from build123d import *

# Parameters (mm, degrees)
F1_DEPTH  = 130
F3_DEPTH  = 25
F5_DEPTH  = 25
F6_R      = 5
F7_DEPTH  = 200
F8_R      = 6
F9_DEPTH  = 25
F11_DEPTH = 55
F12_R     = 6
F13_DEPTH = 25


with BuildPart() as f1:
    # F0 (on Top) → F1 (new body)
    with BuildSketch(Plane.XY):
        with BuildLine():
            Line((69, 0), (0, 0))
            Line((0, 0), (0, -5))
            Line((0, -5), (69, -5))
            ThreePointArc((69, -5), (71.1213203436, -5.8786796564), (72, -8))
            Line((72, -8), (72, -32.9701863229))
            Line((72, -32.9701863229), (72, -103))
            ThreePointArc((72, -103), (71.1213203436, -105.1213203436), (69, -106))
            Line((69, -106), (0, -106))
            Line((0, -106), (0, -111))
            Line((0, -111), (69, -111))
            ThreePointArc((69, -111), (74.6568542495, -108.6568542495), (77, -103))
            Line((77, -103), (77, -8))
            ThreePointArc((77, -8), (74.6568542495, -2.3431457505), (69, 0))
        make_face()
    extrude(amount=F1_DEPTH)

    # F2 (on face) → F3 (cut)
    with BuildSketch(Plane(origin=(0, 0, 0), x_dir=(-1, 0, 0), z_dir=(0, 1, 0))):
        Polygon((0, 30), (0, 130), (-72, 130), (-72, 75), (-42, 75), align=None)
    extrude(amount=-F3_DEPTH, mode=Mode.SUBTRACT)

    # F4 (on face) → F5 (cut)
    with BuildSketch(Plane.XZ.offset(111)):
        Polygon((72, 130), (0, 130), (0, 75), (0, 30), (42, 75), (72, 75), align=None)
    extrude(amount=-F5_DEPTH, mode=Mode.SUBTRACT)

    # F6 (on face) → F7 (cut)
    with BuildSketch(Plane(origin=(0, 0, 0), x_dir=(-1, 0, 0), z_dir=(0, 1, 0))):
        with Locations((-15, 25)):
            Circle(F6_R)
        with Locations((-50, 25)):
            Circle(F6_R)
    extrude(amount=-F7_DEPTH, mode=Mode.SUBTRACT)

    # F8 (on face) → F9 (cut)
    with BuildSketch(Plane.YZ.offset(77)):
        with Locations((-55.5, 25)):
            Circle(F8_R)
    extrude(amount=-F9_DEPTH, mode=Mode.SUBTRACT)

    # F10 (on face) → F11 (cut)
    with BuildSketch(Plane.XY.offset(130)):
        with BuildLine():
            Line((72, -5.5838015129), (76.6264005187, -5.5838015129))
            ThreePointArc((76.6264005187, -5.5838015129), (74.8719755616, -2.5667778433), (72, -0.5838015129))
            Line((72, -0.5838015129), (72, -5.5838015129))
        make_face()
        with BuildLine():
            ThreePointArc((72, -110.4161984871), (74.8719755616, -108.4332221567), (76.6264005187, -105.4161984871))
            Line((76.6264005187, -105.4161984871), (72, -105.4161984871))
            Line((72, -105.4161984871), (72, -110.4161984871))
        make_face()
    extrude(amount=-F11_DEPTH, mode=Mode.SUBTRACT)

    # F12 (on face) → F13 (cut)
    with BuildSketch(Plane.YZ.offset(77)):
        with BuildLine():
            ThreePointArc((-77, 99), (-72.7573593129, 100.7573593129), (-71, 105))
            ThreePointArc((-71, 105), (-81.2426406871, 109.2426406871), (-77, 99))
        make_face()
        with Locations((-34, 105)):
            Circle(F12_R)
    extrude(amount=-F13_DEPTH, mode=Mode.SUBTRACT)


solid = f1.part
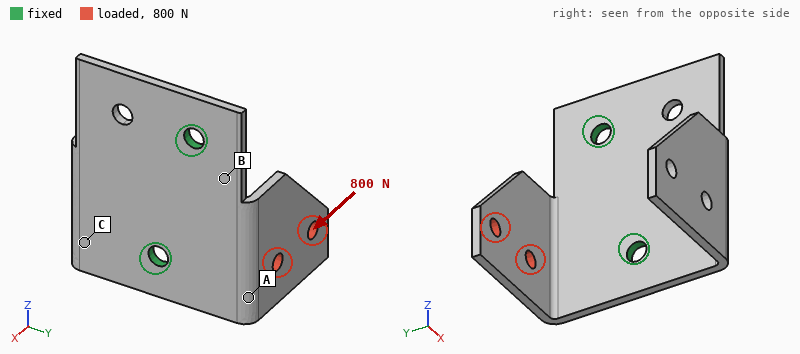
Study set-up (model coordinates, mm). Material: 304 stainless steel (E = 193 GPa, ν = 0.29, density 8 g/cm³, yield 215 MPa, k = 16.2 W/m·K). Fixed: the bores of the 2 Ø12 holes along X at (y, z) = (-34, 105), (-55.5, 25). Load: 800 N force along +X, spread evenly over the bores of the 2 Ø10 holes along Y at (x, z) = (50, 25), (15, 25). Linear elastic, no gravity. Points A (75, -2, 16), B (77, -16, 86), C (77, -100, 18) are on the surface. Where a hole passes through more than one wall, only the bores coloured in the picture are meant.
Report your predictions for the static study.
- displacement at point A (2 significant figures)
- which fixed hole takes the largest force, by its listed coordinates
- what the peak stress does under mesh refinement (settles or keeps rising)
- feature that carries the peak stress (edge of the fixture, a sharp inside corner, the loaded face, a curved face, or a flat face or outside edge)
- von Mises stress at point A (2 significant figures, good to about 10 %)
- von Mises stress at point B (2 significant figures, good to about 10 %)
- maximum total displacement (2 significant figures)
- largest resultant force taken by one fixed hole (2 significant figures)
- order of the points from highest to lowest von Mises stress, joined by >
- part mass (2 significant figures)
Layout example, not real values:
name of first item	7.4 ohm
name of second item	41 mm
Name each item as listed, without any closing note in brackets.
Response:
displacement at point A	0.21 mm
which fixed hole takes the largest force, by its listed coordinates	(-55.5, 25)
what the peak stress does under mesh refinement	keeps rising
feature that carries the peak stress	edge of the fixture
von Mises stress at point A	23 MPa
von Mises stress at point B	43 MPa
maximum total displacement	0.49 mm
largest resultant force taken by one fixed hole	660 N
order of the points from highest to lowest von Mises stress, joined by >	B > A > C
part mass	870 g
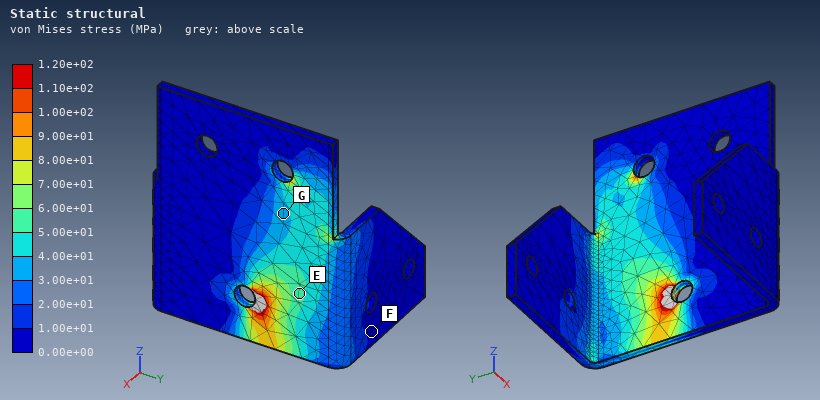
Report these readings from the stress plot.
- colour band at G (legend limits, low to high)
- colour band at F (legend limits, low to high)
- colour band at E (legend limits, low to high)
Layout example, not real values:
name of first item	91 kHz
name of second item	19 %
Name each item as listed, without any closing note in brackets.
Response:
colour band at G	3.00e+01 to 4.00e+01 MPa
colour band at F	0.00e+00 to 1.00e+01 MPa
colour band at E	5.00e+01 to 6.00e+01 MPa
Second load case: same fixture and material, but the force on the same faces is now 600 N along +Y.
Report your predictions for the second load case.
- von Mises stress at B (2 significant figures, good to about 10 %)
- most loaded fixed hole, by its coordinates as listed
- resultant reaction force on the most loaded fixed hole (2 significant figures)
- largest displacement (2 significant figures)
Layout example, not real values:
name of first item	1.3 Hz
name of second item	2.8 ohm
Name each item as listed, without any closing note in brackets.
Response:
von Mises stress at B	50 MPa
most loaded fixed hole, by its coordinates as listed	(-55.5, 25)
resultant reaction force on the most loaded fixed hole	590 N
largest displacement	0.75 mm
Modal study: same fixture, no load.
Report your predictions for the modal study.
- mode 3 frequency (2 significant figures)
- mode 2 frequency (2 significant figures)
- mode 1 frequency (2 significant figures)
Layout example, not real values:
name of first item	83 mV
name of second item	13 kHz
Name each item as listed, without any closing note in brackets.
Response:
mode 3 frequency	720 Hz
mode 2 frequency	470 Hz
mode 1 frequency	430 Hz
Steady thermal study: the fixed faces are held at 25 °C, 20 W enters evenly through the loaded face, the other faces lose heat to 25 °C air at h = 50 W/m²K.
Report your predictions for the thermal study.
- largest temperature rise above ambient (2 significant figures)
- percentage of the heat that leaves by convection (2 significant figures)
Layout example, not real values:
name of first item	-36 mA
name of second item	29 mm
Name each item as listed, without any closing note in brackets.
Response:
largest temperature rise above ambient	74 K
percentage of the heat that leaves by convection	96 %
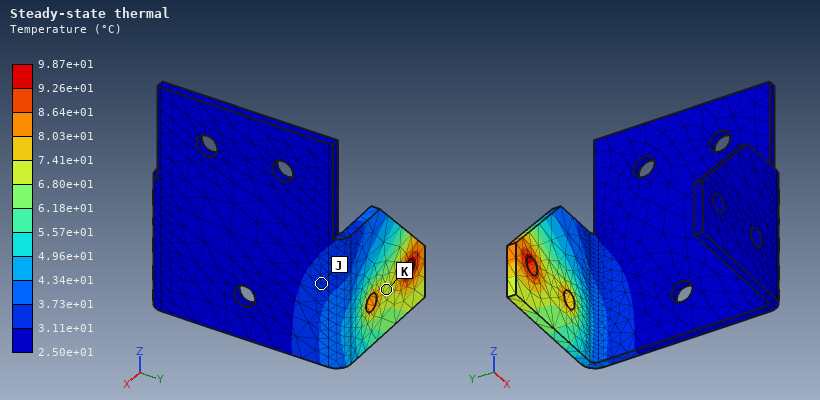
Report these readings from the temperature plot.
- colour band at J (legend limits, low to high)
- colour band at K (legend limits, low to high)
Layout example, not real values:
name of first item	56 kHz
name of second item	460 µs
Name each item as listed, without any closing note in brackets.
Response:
colour band at J	3.11e+01 to 3.73e+01 °C
colour band at K	6.80e+01 to 7.41e+01 °C
